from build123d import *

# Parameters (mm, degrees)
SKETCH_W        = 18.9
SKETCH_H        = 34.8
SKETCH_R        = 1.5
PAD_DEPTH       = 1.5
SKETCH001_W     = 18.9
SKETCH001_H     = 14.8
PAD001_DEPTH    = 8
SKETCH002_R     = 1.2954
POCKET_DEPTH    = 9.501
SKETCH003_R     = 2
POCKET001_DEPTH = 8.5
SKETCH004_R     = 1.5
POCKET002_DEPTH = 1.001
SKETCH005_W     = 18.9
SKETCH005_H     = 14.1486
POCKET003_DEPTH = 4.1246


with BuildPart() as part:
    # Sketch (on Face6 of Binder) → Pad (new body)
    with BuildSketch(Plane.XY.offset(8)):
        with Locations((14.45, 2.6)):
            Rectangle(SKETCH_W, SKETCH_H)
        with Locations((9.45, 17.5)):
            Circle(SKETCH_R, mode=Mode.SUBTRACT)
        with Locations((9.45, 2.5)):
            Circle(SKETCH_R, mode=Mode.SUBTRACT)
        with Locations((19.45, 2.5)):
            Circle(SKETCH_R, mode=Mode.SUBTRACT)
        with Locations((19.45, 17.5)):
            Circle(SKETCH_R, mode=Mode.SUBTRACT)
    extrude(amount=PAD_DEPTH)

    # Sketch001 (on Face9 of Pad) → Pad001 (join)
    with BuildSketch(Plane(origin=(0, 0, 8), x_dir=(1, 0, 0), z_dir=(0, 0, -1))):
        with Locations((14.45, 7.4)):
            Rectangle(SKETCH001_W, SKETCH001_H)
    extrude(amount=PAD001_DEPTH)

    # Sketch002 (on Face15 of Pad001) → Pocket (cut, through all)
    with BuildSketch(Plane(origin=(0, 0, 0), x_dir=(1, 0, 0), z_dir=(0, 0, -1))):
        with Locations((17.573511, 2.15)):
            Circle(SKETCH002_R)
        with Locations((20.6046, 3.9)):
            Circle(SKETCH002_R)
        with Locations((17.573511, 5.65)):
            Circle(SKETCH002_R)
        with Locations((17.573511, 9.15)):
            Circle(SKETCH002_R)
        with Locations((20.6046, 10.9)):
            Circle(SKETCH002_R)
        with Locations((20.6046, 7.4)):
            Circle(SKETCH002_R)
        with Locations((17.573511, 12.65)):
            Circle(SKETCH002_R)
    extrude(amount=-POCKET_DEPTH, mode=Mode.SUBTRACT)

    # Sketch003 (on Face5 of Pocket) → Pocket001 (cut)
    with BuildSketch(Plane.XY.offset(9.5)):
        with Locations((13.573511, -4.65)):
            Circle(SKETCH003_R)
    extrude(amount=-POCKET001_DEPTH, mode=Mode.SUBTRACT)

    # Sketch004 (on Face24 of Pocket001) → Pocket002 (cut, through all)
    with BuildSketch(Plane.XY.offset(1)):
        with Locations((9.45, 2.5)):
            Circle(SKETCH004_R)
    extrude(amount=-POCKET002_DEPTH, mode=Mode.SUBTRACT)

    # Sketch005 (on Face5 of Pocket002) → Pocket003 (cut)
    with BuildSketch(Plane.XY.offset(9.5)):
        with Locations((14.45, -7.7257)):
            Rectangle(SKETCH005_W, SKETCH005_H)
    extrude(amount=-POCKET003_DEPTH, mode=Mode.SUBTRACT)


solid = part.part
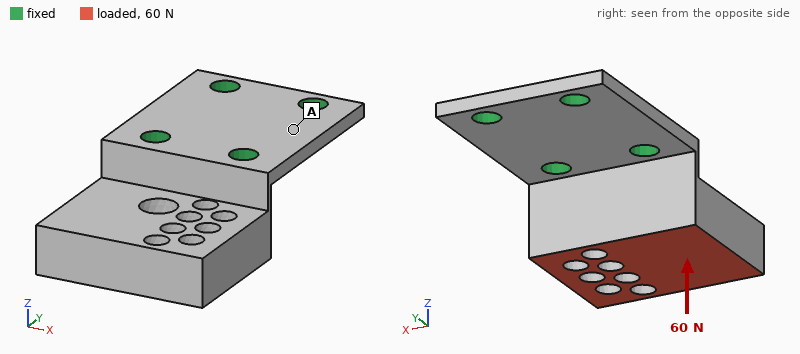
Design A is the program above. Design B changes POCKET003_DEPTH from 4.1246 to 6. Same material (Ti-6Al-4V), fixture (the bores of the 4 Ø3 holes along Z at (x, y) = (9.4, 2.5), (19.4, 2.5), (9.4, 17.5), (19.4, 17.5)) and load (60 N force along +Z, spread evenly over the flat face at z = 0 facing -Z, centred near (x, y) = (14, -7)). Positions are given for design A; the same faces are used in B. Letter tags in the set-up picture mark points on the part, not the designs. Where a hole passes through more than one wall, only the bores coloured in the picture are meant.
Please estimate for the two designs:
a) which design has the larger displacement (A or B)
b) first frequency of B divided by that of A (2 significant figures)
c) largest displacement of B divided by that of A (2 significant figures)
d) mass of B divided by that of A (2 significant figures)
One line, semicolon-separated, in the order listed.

B; 0.99; 1.5; 0.78
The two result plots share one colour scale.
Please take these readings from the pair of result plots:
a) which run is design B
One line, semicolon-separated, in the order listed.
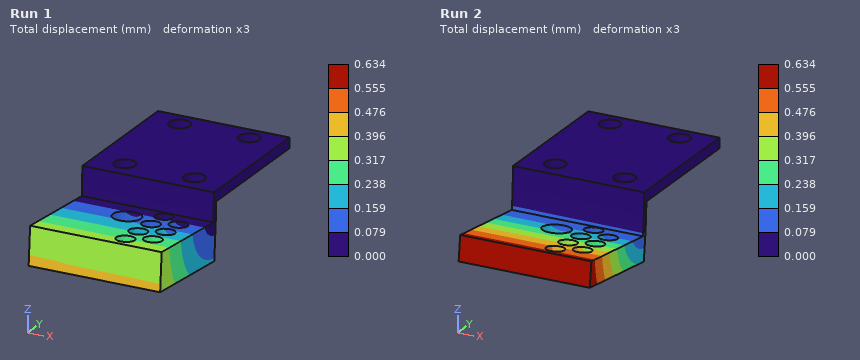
Run 2
